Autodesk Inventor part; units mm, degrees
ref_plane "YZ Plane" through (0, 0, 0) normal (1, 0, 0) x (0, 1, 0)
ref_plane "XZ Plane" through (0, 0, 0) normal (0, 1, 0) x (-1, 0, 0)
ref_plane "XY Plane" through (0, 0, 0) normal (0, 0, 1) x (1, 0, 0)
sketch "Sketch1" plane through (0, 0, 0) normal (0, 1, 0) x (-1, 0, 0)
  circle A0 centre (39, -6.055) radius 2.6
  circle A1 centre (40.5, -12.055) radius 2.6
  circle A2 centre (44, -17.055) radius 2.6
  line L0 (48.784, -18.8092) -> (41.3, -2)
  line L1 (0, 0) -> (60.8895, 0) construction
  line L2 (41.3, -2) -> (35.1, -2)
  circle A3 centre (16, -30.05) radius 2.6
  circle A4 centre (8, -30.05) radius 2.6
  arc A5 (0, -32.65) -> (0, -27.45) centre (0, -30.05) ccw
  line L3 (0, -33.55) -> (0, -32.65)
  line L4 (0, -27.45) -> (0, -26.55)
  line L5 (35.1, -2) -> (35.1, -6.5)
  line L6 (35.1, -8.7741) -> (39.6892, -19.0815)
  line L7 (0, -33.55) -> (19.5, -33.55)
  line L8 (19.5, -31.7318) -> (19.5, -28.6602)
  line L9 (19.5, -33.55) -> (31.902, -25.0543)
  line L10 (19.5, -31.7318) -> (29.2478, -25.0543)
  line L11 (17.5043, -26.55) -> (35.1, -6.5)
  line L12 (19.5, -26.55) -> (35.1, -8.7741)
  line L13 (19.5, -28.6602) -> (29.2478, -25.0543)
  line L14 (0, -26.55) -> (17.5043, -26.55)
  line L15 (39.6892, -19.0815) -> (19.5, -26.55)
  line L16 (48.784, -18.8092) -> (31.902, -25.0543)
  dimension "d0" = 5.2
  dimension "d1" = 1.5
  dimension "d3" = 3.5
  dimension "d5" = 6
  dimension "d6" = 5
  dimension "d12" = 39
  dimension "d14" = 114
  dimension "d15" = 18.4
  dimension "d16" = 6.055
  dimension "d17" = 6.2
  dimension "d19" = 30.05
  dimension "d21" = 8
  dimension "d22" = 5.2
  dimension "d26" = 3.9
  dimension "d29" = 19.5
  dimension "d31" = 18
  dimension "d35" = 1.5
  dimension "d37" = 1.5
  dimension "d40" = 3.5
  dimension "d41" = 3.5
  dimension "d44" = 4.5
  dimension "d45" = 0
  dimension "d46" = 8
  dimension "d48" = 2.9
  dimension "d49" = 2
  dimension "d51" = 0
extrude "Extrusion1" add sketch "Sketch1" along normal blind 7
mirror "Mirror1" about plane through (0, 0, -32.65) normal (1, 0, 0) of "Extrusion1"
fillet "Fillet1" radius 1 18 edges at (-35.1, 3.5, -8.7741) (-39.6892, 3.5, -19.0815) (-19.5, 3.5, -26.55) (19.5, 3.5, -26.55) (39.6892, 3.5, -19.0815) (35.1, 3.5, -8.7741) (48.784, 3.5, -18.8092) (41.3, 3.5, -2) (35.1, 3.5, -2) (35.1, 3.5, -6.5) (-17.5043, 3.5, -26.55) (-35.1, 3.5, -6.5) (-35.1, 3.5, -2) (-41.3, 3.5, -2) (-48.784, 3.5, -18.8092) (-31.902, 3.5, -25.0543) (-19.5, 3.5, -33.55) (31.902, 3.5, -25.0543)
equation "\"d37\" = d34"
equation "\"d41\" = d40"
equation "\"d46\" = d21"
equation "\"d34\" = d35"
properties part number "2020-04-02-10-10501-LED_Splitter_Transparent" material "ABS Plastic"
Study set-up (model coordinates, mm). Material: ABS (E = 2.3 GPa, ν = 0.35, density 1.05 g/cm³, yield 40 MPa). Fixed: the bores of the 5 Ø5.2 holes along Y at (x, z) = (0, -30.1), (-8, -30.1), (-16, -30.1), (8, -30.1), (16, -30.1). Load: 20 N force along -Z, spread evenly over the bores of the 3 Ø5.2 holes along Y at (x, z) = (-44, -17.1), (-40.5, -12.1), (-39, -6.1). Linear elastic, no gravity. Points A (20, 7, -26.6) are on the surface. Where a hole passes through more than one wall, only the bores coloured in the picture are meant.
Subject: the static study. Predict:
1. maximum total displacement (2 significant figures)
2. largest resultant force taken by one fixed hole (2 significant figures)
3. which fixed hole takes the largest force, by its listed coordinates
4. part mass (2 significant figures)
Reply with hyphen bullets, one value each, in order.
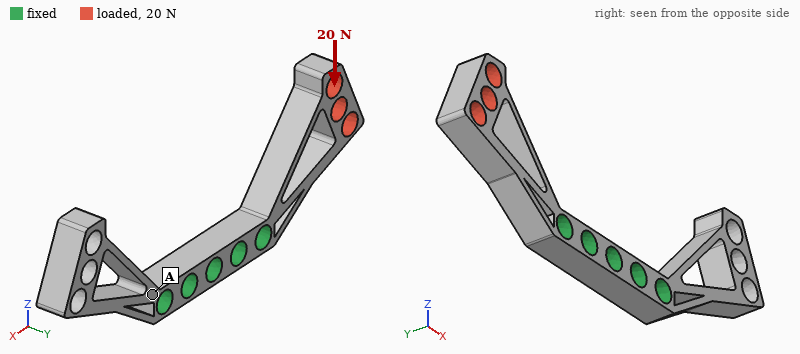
- 0.81 mm
- 21 N
- (-16, -30.1)
- 4.3 g
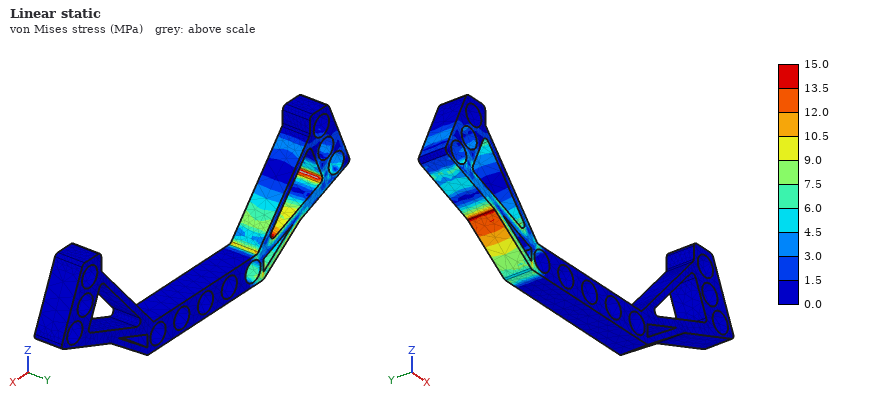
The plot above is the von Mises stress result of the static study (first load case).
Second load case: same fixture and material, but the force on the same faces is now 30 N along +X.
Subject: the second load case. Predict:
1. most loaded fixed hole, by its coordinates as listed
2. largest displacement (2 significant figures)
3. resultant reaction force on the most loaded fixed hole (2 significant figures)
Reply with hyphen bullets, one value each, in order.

- (-16, -30.1)
- 0.92 mm
- 30 N
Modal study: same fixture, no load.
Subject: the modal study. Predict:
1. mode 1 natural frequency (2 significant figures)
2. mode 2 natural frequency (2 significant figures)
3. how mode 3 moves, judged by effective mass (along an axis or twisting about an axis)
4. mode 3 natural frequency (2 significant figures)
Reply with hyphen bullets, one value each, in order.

- 840 Hz
- 840 Hz
- along Y
- 1000 Hz
